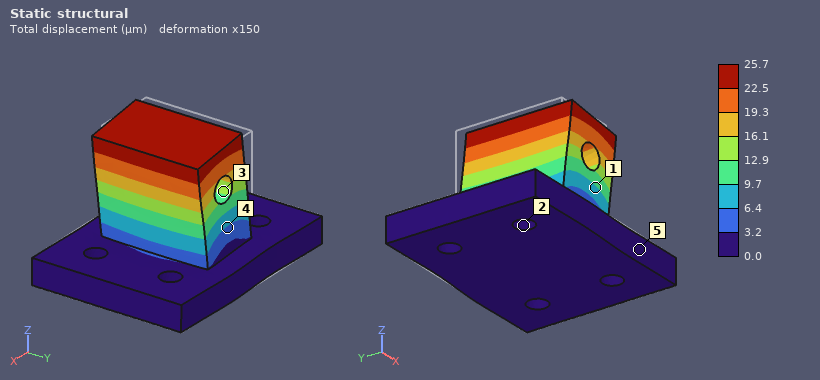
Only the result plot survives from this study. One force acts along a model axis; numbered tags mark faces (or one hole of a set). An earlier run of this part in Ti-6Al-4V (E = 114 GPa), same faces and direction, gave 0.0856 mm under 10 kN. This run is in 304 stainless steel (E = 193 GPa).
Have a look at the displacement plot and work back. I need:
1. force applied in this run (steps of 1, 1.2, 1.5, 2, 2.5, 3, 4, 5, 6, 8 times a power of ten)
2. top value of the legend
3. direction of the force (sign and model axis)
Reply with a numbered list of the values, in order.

1. 5 kN
2. 25.7 µm
3. +X
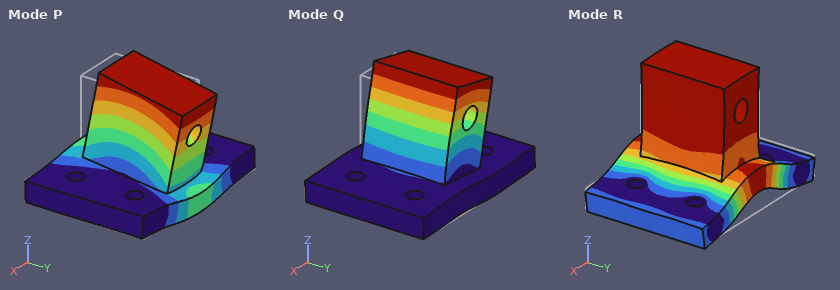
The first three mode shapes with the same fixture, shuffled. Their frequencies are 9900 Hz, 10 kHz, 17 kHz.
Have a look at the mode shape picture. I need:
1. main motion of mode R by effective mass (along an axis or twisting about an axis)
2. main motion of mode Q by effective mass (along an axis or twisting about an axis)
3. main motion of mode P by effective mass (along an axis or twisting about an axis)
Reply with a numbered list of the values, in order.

1. along Z
2. along X
3. along Y
